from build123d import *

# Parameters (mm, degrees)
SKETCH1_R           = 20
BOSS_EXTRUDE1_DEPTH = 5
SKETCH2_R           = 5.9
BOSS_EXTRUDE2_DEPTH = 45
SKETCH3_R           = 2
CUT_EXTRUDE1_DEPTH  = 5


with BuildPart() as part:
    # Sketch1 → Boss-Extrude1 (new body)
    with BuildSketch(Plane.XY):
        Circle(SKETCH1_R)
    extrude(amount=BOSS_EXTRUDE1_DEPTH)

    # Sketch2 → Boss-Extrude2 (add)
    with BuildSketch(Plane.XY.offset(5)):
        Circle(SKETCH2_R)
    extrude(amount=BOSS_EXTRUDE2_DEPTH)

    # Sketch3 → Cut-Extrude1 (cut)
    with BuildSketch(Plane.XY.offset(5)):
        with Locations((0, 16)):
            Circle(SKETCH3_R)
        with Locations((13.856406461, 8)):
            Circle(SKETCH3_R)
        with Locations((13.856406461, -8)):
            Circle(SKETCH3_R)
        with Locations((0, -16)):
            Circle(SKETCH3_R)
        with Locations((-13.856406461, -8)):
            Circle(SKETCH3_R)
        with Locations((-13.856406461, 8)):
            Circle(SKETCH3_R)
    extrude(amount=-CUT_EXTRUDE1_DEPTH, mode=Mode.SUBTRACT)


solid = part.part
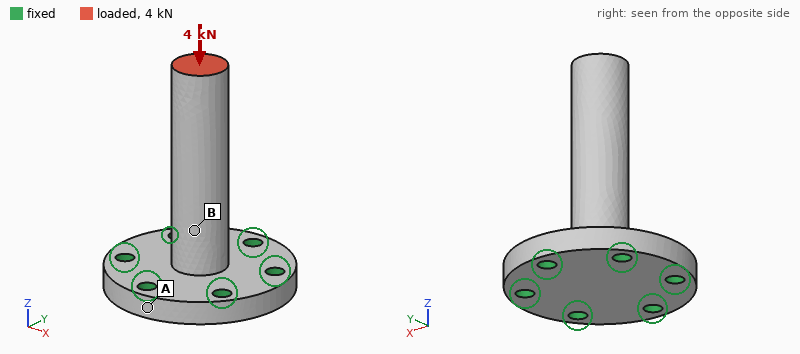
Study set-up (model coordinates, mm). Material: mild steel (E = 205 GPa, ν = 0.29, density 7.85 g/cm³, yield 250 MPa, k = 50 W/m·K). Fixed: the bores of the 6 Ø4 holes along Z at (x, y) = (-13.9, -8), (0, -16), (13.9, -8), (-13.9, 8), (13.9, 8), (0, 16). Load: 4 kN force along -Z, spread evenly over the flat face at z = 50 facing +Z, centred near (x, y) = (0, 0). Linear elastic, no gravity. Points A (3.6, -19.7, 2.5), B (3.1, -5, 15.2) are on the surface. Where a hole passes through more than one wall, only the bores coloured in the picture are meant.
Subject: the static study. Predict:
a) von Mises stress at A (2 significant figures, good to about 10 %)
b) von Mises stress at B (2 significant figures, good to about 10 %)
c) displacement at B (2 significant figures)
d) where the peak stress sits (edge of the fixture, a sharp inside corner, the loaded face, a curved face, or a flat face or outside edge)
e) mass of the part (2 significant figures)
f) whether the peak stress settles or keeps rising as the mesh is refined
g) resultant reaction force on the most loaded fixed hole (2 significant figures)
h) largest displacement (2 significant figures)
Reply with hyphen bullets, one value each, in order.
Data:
- 14 MPa
- 36 MPa
- 7.6 µm
- edge of the fixture
- 85 g
- keeps rising
- 690 N
- 14 µm
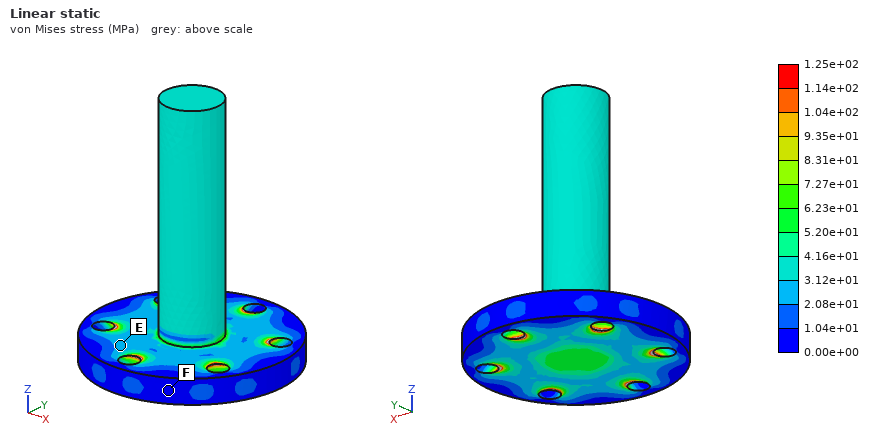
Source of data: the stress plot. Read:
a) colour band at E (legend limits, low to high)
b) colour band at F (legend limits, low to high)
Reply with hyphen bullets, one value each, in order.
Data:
- 2.08e+01 to 3.12e+01 MPa
- 0.00e+00 to 1.04e+01 MPa
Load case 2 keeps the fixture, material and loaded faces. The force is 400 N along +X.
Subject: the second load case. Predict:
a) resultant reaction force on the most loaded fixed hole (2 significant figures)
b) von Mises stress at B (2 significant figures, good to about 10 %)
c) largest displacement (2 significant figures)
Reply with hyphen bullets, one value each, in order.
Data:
- 460 N
- 45 MPa
- 91 µm
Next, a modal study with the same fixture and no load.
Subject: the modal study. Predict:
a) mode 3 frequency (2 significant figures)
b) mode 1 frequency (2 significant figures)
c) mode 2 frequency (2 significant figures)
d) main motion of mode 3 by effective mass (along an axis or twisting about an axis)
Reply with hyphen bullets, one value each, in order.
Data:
- 16 kHz
- 3300 Hz
- 3300 Hz
- along Z
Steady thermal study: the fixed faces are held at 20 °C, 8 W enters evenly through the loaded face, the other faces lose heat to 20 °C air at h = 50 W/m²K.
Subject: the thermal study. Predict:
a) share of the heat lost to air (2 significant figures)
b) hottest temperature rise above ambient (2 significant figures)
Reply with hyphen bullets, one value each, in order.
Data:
- 33 %
- 58 K
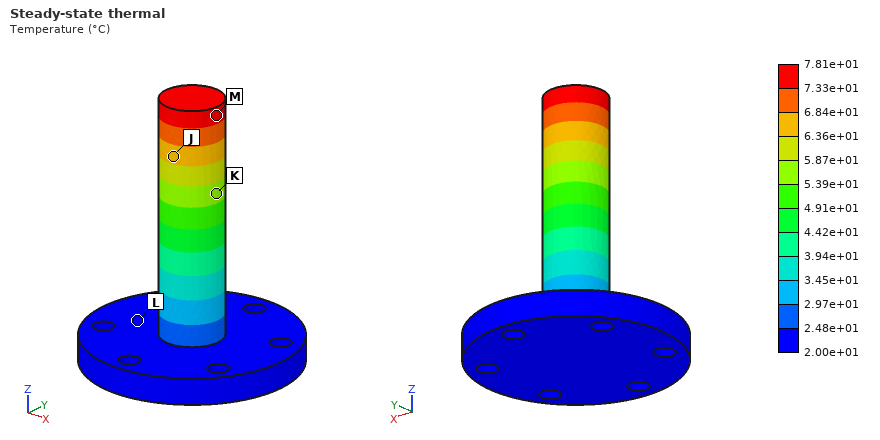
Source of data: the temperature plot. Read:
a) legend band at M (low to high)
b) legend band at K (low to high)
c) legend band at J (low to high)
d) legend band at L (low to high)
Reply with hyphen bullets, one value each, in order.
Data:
- 7.33e+01 to 7.81e+01 °C
- 5.39e+01 to 5.87e+01 °C
- 6.36e+01 to 6.84e+01 °C
- 2.00e+01 to 2.48e+01 °C
